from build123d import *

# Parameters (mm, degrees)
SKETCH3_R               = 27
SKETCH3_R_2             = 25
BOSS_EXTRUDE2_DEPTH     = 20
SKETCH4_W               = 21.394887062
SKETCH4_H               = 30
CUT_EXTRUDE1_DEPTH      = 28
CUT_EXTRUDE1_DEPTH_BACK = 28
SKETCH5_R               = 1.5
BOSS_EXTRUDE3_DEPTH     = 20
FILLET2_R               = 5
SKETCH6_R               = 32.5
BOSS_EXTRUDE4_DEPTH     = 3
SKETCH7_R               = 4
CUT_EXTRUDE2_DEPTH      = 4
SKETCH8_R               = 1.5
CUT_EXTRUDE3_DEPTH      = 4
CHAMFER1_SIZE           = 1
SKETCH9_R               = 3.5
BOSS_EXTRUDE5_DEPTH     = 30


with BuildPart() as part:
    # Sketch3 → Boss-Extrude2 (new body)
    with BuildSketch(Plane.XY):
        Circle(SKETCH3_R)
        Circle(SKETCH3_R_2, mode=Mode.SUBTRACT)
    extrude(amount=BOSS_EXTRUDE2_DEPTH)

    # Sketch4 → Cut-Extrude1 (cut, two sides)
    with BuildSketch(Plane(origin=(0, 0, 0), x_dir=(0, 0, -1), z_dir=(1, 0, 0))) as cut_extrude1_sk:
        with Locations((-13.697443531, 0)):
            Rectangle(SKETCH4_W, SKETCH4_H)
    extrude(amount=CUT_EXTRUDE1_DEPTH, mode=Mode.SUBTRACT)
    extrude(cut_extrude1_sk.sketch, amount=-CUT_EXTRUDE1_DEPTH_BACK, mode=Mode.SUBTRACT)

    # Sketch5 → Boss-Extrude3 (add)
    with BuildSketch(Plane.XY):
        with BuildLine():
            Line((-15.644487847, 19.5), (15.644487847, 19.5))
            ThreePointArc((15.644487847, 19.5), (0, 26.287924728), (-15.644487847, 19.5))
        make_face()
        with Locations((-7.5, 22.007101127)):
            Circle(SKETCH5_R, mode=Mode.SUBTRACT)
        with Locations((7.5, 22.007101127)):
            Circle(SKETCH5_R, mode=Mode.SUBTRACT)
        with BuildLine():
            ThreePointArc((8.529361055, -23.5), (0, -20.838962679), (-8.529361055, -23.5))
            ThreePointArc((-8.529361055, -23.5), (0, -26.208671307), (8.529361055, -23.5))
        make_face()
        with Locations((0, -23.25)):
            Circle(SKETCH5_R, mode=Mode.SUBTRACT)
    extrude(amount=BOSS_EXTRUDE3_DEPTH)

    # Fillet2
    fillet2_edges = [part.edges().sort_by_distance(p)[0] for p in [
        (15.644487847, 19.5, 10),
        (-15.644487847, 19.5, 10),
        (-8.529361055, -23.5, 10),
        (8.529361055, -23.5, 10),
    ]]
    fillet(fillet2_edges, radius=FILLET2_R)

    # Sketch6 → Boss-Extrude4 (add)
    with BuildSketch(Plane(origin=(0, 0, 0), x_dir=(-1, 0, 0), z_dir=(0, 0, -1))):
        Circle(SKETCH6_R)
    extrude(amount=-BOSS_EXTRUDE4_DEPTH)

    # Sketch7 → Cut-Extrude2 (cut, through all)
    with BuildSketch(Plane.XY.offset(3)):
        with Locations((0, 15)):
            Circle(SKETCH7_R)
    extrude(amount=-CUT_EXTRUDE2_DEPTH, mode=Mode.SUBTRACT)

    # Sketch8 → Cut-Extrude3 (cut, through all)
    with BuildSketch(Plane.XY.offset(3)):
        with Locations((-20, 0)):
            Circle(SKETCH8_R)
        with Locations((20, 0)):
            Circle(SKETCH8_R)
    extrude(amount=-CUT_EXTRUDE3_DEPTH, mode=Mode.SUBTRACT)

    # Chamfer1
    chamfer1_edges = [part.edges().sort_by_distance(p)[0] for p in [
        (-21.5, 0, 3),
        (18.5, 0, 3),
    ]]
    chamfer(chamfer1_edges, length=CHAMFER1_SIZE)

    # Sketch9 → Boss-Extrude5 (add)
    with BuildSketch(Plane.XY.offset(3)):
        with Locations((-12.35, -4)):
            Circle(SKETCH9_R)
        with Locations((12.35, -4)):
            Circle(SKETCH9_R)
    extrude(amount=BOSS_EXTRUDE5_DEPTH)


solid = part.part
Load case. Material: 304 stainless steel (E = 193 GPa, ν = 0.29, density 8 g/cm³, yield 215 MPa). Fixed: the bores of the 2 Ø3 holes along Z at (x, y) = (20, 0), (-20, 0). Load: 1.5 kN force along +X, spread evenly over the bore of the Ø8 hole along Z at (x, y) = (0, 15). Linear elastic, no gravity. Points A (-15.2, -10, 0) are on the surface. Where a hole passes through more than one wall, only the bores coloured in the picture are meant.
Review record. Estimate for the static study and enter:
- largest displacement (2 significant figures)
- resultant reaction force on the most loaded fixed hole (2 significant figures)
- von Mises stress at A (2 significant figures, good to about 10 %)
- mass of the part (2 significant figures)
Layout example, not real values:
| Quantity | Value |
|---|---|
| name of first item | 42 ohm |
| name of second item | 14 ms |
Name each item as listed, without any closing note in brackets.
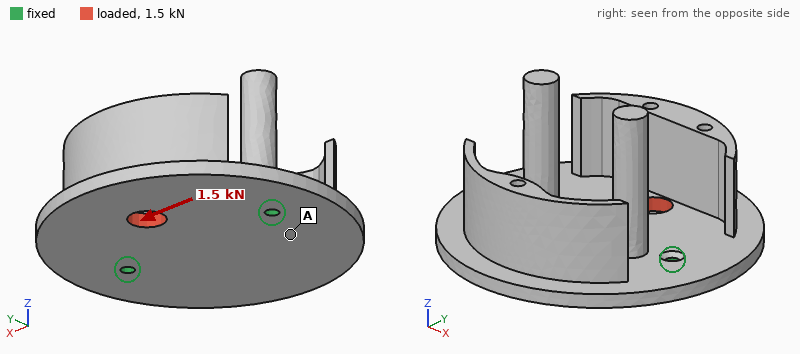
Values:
| Quantity | Value |
|---|---|
| largest displacement | 4.1 µm |
| resultant reaction force on the most loaded fixed hole | 930 N |
| von Mises stress at A | 4.3 MPa |
| mass of the part | 140 g |
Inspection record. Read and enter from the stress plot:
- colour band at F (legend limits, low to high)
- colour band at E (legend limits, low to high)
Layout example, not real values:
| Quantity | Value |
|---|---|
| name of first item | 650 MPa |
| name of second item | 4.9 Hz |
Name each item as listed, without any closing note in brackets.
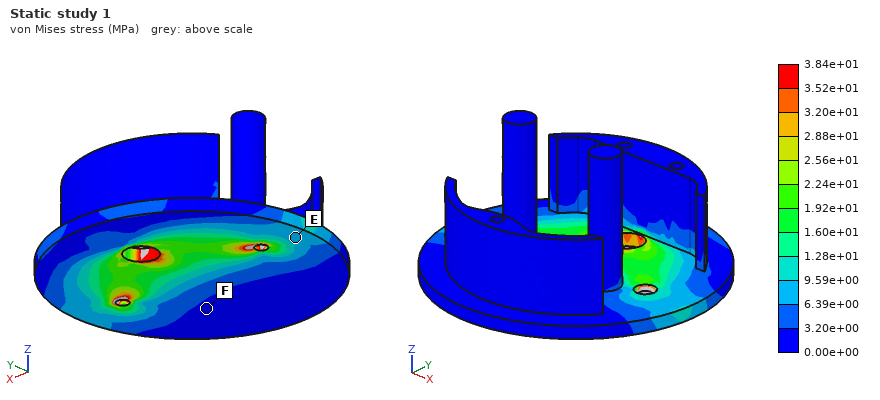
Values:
| Quantity | Value |
|---|---|
| colour band at F | 0.00e+00 to 3.20e+00 MPa |
| colour band at E | 6.39e+00 to 9.59e+00 MPa |
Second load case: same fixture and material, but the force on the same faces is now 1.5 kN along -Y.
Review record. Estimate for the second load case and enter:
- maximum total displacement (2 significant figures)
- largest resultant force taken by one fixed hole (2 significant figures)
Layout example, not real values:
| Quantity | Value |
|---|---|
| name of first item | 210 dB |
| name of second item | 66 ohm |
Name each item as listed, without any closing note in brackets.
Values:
| Quantity | Value |
|---|---|
| maximum total displacement | 5.2 µm |
| largest resultant force taken by one fixed hole | 760 N |
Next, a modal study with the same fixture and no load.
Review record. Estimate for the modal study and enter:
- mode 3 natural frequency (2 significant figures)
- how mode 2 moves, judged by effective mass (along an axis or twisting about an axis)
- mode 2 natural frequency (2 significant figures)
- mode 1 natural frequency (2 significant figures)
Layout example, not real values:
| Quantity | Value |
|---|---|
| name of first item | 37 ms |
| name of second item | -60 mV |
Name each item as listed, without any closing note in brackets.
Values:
| Quantity | Value |
|---|---|
| mode 3 natural frequency | 3300 Hz |
| how mode 2 moves, judged by effective mass | along Z |
| mode 2 natural frequency | 1700 Hz |
| mode 1 natural frequency | 1200 Hz |
